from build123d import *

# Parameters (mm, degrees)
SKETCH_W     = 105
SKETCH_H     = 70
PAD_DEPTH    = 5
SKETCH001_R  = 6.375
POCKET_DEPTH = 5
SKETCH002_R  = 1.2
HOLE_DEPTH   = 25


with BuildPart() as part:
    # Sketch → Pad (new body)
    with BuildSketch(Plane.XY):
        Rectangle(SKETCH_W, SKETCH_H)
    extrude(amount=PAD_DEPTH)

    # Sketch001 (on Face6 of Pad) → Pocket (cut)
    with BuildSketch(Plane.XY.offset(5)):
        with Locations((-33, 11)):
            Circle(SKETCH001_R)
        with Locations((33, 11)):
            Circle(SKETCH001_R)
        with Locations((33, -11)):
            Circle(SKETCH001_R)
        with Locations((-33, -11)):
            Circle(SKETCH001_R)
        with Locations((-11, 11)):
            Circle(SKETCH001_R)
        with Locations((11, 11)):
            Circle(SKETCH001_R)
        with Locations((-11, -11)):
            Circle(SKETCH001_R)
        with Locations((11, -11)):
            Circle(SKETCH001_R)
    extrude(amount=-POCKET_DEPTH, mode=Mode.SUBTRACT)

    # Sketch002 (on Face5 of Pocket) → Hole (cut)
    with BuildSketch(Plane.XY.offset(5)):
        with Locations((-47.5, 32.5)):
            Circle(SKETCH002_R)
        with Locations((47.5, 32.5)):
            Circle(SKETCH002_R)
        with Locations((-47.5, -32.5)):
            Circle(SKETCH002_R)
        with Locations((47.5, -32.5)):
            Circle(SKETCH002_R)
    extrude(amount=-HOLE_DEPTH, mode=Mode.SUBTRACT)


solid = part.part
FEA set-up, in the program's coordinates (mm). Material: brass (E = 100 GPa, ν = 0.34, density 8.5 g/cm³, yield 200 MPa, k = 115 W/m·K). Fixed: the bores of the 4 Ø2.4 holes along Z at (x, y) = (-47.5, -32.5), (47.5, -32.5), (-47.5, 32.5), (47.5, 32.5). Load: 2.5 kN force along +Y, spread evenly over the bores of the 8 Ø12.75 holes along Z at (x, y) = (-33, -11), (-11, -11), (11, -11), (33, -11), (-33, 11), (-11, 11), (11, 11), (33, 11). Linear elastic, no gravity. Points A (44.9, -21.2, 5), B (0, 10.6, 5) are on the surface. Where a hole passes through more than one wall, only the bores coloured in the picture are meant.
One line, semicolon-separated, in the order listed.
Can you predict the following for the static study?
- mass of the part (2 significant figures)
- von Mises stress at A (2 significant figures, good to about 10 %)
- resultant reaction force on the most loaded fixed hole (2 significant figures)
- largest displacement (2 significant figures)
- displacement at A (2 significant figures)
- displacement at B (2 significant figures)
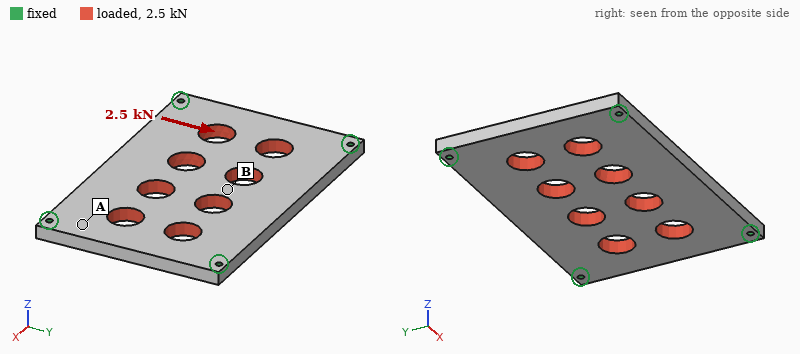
270 g; 7.3 MPa; 730 N; 7.1 µm; 1.5 µm; 7.0 µm
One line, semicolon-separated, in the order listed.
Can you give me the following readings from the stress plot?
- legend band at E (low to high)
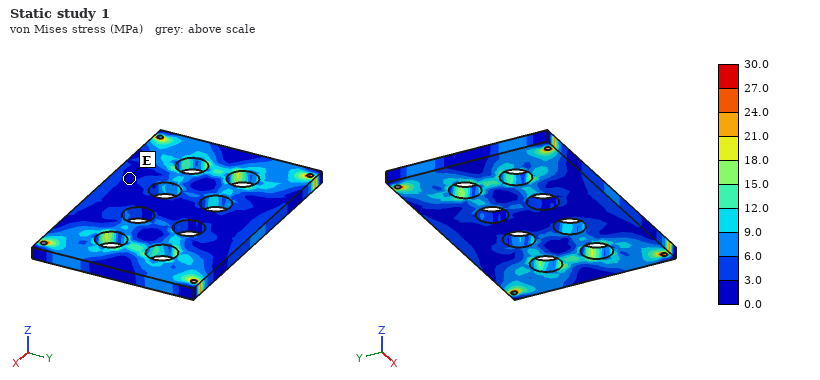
0.0 to 3.0 MPa
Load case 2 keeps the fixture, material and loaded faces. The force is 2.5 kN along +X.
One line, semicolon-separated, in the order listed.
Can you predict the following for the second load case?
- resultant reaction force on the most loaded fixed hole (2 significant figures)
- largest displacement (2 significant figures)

670 N; 4.7 µm
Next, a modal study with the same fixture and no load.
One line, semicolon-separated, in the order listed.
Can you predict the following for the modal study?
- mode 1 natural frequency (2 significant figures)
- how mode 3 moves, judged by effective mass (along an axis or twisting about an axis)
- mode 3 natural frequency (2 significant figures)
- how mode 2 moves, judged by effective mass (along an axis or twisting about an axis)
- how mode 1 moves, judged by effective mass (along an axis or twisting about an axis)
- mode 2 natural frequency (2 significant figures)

1400 Hz; twisting about Y; 3200 Hz; twisting about X; along Z; 2300 Hz
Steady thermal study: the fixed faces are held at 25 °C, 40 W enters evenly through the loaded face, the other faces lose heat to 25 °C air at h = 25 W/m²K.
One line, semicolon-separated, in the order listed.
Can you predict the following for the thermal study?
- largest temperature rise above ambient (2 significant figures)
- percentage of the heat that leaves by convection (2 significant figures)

26 K; 15 %
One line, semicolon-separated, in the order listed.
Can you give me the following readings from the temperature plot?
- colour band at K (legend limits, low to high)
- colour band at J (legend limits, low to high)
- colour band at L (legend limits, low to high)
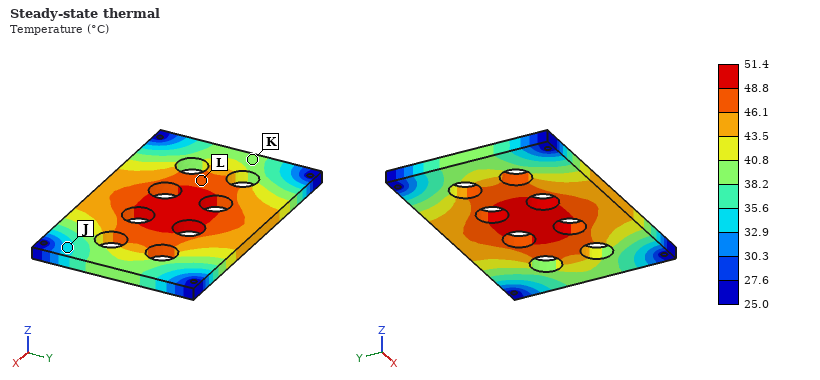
38.2 to 40.8 °C; 32.9 to 35.6 °C; 46.1 to 48.8 °C
